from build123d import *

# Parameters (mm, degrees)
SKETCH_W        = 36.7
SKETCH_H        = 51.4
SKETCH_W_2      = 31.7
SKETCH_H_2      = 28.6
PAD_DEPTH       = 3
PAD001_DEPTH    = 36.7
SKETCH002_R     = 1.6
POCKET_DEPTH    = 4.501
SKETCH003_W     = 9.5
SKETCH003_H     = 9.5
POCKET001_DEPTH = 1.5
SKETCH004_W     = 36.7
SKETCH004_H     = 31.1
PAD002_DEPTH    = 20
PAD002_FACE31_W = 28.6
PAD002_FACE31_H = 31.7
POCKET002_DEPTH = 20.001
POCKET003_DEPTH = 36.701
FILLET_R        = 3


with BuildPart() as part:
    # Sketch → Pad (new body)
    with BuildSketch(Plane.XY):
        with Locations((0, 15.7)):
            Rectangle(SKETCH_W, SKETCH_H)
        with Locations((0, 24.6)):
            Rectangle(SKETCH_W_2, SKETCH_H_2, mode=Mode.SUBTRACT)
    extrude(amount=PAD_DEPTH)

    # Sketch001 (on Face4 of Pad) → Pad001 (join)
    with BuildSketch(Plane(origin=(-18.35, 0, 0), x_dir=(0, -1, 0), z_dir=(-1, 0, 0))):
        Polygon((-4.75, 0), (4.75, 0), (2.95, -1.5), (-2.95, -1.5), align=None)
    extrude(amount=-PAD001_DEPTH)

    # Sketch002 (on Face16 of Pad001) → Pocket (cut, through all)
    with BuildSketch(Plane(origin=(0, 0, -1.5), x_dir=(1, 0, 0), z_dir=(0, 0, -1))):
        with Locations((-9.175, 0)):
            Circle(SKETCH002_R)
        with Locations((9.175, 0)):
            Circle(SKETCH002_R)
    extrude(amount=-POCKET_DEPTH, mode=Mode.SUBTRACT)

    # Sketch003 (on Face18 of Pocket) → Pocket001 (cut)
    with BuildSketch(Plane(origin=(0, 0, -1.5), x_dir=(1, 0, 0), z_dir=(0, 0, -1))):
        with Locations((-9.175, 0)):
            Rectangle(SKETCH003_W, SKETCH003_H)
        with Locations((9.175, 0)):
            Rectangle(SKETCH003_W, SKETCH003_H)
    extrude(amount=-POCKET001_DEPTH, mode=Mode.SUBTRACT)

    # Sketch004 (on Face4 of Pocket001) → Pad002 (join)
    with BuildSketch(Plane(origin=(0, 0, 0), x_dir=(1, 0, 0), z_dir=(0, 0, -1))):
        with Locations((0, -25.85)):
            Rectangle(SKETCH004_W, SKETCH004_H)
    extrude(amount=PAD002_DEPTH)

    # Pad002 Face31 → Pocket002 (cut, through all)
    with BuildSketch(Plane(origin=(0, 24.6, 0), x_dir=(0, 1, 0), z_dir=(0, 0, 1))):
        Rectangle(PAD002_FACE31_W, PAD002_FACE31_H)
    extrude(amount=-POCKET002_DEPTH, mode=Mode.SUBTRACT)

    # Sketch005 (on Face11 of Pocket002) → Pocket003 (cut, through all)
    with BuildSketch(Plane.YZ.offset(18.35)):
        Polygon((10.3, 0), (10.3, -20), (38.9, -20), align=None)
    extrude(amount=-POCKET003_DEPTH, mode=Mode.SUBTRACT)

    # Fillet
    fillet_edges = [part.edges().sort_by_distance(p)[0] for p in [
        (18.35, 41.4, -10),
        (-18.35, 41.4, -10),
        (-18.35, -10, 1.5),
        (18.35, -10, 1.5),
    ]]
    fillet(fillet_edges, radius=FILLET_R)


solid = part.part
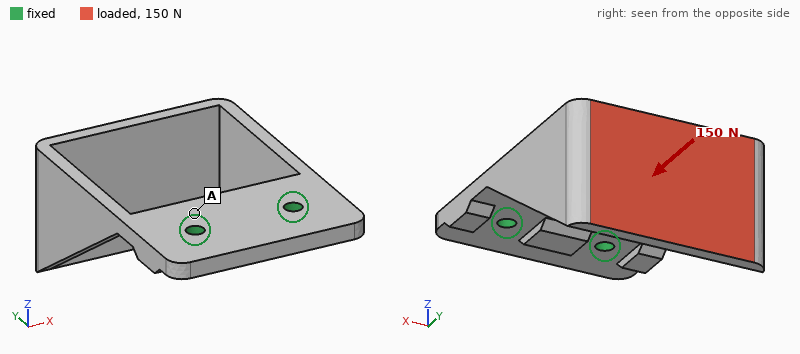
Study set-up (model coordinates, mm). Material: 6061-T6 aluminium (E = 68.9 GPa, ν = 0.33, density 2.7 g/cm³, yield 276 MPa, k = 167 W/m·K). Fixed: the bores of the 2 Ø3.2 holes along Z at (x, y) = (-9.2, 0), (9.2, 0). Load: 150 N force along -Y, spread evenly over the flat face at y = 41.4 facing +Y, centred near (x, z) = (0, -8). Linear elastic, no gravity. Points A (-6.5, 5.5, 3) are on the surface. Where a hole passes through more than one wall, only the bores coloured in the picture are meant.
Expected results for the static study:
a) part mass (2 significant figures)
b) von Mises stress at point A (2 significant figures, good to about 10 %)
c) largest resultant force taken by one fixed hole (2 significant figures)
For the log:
17 g
17 MPa
75 N
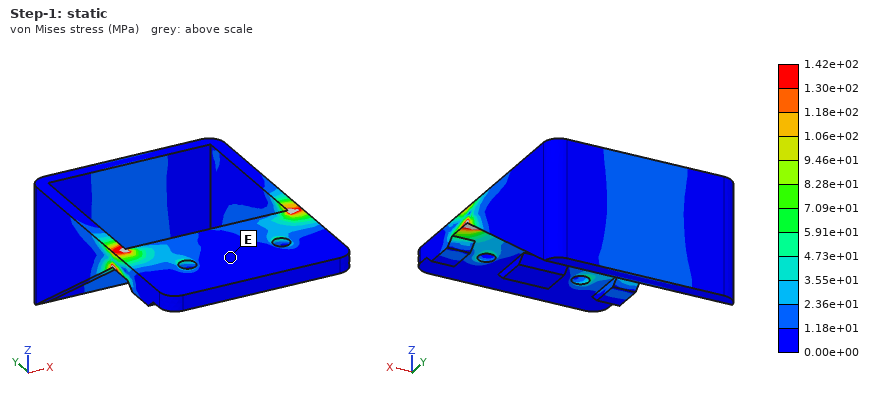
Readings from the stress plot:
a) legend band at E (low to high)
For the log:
0.00e+00 to 1.18e+01 MPa
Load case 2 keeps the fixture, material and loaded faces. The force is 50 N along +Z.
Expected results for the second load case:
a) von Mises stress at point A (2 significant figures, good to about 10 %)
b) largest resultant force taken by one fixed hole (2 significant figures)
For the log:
23 MPa
28 N
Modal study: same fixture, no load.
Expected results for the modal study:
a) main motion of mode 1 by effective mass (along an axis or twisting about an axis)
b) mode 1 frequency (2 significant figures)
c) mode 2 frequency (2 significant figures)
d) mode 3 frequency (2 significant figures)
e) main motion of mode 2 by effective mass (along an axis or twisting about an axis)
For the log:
along Z
600 Hz
1100 Hz
1700 Hz
along X
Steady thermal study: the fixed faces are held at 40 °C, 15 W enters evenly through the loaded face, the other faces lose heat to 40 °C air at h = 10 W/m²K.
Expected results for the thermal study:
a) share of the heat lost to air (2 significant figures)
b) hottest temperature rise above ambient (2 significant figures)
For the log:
13 %
81 K
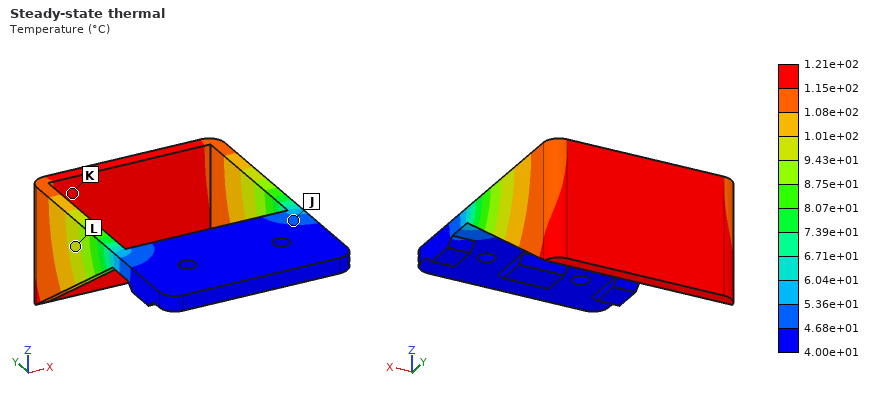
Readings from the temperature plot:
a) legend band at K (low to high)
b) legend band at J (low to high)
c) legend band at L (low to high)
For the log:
1.15e+02 to 1.21e+02 °C
4.68e+01 to 5.36e+01 °C
9.43e+01 to 1.01e+02 °C
